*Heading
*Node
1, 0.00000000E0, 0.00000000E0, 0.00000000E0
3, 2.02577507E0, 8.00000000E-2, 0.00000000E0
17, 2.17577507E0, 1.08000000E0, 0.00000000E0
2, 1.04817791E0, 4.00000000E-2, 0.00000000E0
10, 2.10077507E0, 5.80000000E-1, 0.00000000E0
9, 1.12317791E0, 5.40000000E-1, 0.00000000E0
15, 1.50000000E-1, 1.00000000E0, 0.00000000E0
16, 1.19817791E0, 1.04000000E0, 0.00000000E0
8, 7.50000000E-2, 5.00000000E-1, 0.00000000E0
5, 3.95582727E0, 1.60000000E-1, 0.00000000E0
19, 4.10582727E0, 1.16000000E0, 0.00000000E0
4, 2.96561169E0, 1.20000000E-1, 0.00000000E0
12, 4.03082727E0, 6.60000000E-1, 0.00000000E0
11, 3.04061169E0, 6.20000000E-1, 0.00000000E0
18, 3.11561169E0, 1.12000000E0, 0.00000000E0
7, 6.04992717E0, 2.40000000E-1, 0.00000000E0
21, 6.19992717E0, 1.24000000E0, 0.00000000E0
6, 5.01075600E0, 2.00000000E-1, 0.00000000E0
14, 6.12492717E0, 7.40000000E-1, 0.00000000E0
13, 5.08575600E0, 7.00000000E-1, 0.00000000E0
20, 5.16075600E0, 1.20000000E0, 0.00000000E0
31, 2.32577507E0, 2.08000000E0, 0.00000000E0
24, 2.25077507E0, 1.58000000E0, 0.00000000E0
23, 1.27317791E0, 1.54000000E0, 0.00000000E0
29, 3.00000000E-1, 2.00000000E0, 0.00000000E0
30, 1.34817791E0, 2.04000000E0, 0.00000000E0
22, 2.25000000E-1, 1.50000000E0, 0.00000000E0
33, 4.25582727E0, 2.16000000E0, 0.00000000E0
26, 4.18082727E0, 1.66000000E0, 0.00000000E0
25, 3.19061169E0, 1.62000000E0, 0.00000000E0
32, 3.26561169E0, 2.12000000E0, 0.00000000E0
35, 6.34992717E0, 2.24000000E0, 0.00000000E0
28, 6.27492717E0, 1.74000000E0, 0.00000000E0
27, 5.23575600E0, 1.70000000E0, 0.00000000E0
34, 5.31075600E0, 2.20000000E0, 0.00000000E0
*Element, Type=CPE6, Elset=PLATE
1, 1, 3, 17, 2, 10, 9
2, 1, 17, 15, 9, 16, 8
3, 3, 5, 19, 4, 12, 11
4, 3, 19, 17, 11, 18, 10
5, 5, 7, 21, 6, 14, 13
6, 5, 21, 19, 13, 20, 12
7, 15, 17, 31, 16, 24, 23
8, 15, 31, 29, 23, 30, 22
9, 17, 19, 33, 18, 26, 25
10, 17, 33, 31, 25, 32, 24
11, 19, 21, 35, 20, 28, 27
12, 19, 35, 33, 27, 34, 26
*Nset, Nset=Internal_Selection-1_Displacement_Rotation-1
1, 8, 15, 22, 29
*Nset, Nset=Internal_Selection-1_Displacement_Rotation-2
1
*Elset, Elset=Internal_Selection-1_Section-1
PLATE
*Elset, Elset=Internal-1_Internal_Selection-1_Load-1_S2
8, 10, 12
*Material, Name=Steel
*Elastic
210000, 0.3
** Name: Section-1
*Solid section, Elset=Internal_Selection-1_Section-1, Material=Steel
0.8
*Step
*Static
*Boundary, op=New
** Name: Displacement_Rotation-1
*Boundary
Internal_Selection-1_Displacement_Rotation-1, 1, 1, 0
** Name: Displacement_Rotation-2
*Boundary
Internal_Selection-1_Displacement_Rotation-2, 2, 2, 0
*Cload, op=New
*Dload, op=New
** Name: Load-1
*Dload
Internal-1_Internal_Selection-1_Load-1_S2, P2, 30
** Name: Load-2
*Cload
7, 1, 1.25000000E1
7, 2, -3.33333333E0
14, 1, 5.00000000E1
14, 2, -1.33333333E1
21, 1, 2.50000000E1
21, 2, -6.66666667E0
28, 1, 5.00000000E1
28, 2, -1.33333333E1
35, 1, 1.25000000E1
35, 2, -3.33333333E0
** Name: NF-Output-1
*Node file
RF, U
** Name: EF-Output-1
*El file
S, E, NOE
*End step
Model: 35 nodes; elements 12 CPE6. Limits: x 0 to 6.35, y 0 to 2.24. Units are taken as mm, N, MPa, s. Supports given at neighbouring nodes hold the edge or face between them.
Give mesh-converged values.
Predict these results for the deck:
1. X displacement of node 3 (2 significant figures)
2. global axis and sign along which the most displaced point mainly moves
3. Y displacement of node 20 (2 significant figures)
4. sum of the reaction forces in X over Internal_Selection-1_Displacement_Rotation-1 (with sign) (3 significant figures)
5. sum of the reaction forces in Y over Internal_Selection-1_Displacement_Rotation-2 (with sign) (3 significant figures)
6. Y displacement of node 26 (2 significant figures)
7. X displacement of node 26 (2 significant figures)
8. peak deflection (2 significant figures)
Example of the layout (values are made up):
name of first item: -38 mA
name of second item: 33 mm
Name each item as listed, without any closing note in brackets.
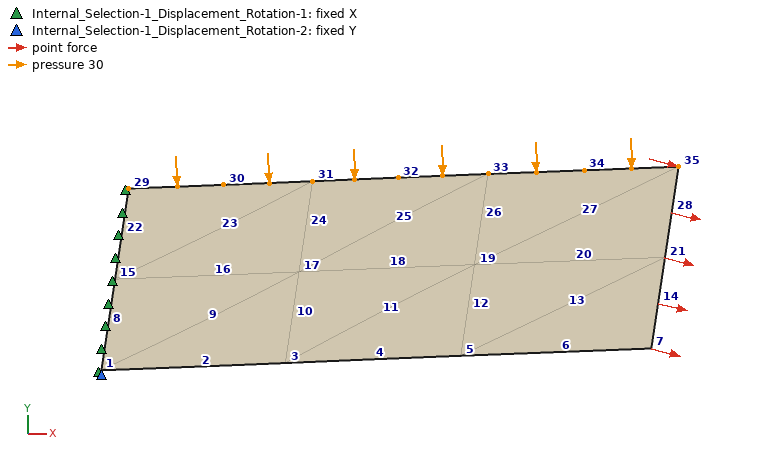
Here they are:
X displacement of node 3: -0.0075 mm
global axis and sign along which the most displaced point mainly moves: -Y
Y displacement of node 20: -0.056 mm
sum of the reaction forces in X over Internal_Selection-1_Displacement_Rotation-1 (with sign): -156 N
sum of the reaction forces in Y over Internal_Selection-1_Displacement_Rotation-2 (with sign): 185 N
Y displacement of node 26: -0.042 mm
X displacement of node 26: 0.0098 mm
peak deflection: 0.077 mm
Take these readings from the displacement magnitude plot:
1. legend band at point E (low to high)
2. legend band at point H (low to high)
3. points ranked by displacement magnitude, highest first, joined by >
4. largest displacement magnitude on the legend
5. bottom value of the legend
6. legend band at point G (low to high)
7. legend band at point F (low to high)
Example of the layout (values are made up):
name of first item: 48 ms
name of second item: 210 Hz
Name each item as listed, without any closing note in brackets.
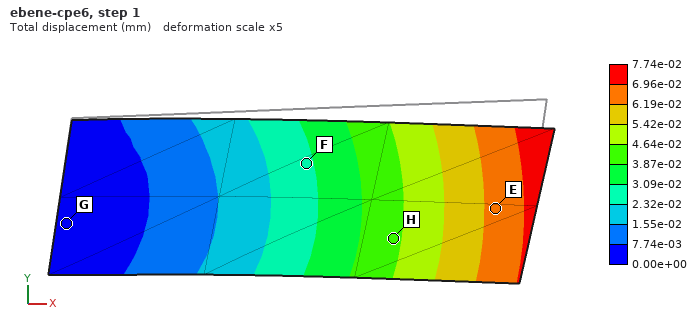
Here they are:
legend band at point E: 6.19e-02 to 6.96e-02 mm
legend band at point H: 3.87e-02 to 4.64e-02 mm
points ranked by displacement magnitude, highest first, joined by >: E > H > F > G
largest displacement magnitude on the legend: 7.74e-02 mm
bottom value of the legend: 0.00e+00 mm
legend band at point G: 0.00e+00 to 7.74e-03 mm
legend band at point F: 2.32e-02 to 3.09e-02 mm
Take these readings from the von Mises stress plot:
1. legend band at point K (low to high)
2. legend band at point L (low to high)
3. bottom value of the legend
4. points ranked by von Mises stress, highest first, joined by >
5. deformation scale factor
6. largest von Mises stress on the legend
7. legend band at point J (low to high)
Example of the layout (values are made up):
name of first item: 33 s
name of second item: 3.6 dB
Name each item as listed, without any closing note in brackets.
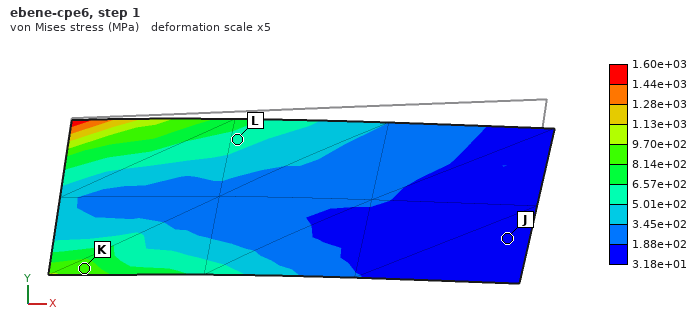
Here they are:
legend band at point K: 8.14e+02 to 9.70e+02 MPa
legend band at point L: 5.01e+02 to 6.57e+02 MPa
bottom value of the legend: 3.18e+01 MPa
points ranked by von Mises stress, highest first, joined by >: K > L > J
deformation scale factor: 5
largest von Mises stress on the legend: 1.60e+03 MPa
legend band at point J: 3.18e+01 to 1.88e+02 MPa
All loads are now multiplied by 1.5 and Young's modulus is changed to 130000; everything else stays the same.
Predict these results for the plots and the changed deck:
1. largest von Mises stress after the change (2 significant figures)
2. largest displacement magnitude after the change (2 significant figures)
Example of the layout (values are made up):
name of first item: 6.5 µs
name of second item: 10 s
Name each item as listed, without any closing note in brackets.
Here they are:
largest von Mises stress after the change: 2400 MPa
largest displacement magnitude after the change: 0.19 mm
